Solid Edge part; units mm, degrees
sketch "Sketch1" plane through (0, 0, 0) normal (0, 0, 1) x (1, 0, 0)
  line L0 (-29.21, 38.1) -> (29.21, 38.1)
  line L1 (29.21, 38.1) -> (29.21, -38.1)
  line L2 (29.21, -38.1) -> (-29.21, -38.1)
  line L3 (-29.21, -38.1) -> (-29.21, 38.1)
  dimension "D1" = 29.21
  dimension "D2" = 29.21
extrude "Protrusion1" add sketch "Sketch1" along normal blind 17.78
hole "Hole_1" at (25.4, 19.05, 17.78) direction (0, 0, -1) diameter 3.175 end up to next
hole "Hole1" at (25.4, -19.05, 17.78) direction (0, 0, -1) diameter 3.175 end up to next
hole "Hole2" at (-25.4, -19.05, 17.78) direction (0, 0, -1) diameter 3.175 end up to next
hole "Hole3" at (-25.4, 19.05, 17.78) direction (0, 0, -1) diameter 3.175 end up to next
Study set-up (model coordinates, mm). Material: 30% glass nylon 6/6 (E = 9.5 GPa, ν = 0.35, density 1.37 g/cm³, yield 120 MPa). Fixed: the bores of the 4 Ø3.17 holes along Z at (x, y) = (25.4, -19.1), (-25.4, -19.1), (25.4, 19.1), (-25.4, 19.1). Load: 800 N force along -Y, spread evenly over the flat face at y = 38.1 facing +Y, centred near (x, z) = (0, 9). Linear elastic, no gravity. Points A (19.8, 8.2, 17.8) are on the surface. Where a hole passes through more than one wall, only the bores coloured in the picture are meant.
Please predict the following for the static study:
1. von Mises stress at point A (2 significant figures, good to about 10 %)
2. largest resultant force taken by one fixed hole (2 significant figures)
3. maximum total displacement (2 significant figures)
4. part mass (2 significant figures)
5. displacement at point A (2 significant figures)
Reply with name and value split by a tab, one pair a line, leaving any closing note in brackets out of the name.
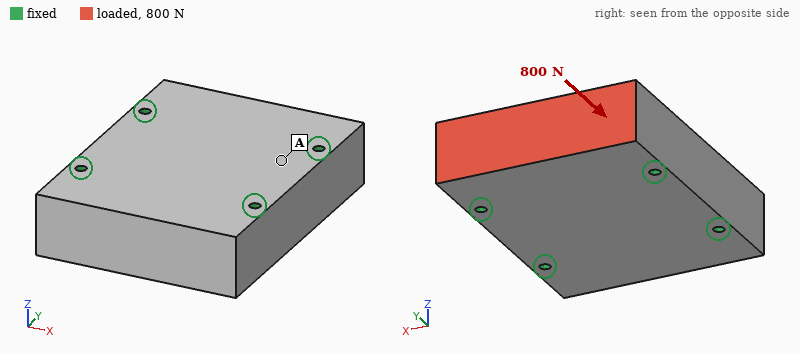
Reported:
von Mises stress at point A	0.46 MPa
largest resultant force taken by one fixed hole	300 N
maximum total displacement	3.3 µm
part mass	110 g
displacement at point A	0.91 µm
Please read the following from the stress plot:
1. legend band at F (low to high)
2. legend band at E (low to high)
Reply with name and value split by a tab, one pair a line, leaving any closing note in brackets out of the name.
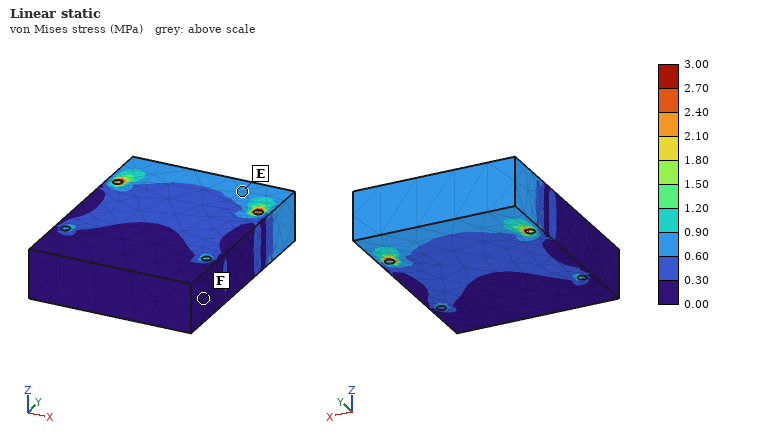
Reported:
legend band at F	0.00 to 0.30 MPa
legend band at E	0.60 to 0.90 MPa
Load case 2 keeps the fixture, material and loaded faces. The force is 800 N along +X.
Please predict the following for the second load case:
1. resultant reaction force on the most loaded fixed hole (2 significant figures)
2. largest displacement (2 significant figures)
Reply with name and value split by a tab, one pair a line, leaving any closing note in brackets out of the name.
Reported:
resultant reaction force on the most loaded fixed hole	470 N
largest displacement	9.0 µm
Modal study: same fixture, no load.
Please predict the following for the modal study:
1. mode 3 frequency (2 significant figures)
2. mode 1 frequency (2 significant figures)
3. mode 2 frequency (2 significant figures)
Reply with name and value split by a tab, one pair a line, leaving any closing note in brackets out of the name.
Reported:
mode 3 frequency	11 kHz
mode 1 frequency	7700 Hz
mode 2 frequency	7800 Hz
